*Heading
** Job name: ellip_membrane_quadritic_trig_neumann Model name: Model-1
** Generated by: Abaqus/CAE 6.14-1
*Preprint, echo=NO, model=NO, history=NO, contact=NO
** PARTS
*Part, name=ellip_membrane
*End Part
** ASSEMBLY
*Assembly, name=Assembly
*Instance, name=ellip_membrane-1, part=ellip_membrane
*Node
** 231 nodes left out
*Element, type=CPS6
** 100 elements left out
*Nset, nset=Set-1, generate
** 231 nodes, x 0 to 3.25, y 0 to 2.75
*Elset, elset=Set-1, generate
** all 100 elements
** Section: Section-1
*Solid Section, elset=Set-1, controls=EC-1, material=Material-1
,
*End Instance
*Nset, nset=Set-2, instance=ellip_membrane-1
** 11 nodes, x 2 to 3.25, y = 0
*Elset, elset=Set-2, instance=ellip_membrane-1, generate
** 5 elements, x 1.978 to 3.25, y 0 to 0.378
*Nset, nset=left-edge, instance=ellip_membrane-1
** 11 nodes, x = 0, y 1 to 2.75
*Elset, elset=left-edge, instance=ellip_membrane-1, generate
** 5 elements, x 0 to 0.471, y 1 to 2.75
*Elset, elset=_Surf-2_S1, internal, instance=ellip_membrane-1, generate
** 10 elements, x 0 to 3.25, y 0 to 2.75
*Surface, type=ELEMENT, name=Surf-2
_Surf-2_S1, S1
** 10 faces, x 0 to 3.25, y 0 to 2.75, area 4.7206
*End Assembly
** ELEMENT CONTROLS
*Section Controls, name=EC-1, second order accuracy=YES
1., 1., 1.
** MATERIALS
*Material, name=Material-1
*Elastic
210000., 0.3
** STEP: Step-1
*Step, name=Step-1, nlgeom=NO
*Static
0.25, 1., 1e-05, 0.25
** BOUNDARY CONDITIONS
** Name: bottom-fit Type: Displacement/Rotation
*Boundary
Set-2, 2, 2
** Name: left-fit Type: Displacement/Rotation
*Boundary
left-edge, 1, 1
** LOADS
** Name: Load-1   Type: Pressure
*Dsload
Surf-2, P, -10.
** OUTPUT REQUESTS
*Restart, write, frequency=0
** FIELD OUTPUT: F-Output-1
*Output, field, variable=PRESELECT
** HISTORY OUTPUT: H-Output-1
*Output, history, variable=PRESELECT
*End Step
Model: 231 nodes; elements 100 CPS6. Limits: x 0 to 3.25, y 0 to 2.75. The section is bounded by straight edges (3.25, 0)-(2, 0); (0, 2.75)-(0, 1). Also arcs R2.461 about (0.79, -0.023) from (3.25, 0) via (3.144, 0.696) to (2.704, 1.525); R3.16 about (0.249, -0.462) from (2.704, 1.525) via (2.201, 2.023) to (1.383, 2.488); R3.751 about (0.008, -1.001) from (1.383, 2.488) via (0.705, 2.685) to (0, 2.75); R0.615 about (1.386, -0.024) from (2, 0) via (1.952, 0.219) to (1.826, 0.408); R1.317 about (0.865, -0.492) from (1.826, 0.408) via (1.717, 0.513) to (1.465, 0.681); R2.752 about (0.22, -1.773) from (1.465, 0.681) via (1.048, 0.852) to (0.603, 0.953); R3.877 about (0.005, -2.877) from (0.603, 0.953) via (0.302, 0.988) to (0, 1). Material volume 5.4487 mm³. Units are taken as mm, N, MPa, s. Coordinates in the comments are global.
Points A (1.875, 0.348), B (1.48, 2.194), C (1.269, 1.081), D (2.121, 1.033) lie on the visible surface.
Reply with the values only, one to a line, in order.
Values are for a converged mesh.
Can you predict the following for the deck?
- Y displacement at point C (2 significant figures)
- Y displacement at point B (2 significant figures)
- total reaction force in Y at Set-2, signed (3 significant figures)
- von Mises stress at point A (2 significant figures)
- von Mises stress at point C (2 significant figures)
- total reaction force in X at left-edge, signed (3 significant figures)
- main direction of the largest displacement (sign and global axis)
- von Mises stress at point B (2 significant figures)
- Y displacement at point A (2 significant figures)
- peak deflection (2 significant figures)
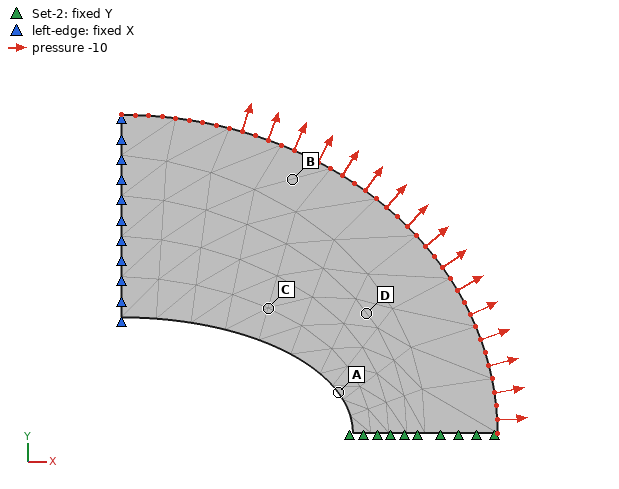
3.9e-04 mm
3.8e-04 mm
-32.5 N
59 MPa
15 MPa
-27.5 N
+Y
22 MPa
1.6e-04 mm
5.5e-04 mm
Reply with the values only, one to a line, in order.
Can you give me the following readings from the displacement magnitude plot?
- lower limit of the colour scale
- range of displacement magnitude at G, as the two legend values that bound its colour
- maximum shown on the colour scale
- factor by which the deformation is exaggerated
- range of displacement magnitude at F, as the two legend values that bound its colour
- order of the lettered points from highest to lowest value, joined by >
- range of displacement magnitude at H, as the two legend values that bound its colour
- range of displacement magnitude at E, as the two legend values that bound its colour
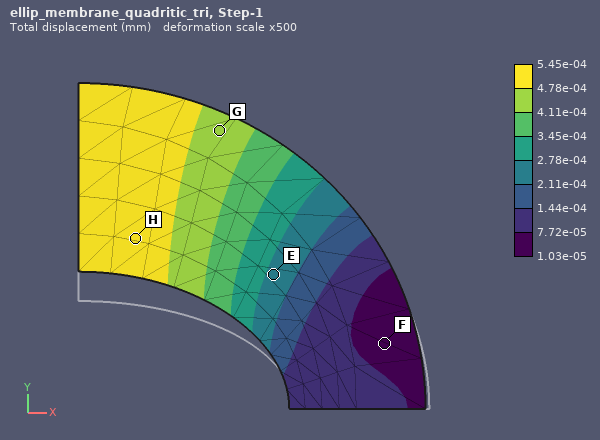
1.03e-05 mm
4.11e-04 to 4.78e-04 mm
5.45e-04 mm
500
1.03e-05 to 7.72e-05 mm
H > G > E > F
4.78e-04 to 5.45e-04 mm
2.11e-04 to 2.78e-04 mm
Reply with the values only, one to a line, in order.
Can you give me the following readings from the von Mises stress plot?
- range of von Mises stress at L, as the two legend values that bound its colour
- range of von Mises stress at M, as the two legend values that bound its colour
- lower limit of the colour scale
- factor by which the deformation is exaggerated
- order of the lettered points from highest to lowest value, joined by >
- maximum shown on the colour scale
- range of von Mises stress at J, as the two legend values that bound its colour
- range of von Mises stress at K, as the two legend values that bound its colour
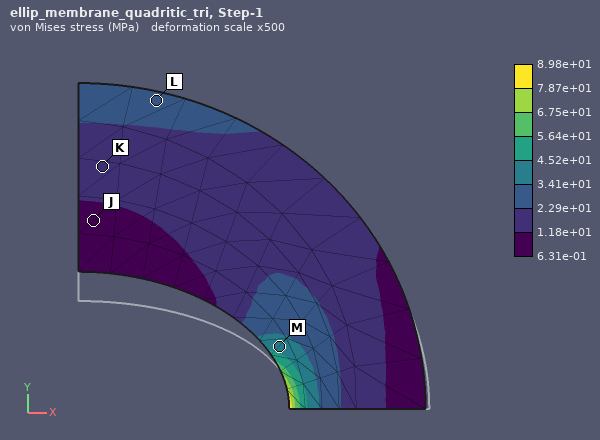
2.29e+01 to 3.41e+01 MPa
3.41e+01 to 4.52e+01 MPa
6.31e-01 MPa
500
M > L > K > J
8.98e+01 MPa
6.31e-01 to 1.18e+01 MPa
1.18e+01 to 2.29e+01 MPa
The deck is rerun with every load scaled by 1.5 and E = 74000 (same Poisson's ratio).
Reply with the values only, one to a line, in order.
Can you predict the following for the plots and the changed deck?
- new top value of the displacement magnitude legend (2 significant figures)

0.0023 mm
